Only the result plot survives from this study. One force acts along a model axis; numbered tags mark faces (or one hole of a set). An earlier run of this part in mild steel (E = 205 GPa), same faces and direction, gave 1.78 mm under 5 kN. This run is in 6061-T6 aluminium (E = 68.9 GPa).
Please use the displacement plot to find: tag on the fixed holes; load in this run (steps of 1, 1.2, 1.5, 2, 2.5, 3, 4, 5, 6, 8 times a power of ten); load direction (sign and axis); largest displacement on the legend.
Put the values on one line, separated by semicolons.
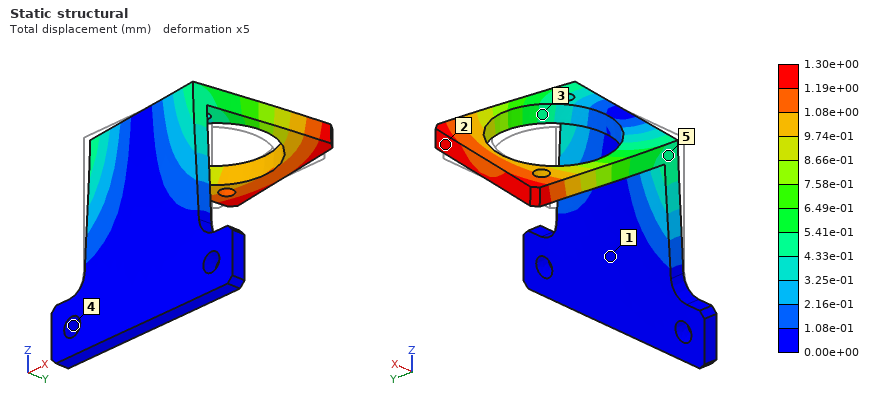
4; 1.2 kN; +X; 1.30e+00 mm
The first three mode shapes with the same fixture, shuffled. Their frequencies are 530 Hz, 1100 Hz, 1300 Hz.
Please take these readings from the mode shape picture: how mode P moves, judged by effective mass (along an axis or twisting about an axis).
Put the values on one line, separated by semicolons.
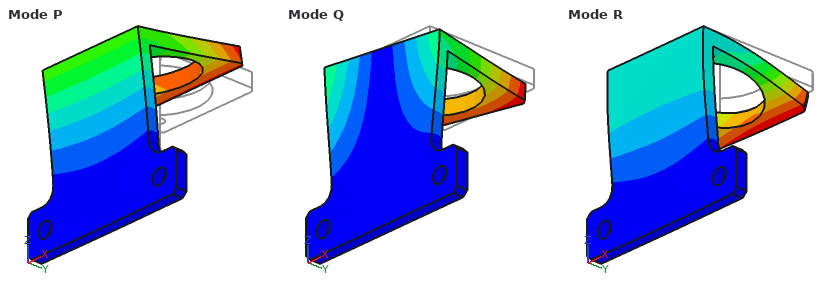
along Y
